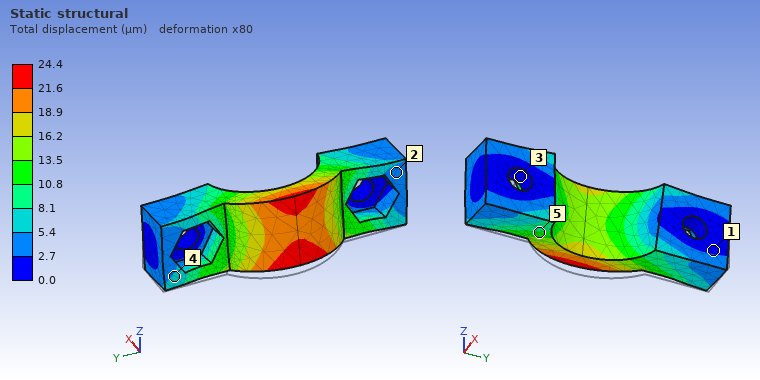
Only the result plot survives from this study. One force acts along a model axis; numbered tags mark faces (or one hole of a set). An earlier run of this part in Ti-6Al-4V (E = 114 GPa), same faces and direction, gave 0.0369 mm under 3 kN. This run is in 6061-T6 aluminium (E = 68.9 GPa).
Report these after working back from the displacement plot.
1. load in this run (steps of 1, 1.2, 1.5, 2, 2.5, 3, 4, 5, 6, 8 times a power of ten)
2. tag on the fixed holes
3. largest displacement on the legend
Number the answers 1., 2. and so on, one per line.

1. 1.2 kN
2. 3
3. 24.4 µm
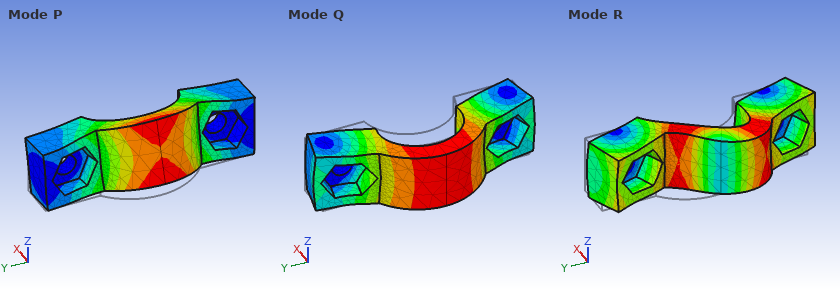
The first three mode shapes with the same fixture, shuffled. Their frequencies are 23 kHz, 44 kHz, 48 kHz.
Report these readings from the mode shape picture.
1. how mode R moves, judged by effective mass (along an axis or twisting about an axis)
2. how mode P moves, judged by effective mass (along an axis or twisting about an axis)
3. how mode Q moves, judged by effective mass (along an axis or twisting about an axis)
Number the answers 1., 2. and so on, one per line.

1. along Y
2. along Z
3. along X
